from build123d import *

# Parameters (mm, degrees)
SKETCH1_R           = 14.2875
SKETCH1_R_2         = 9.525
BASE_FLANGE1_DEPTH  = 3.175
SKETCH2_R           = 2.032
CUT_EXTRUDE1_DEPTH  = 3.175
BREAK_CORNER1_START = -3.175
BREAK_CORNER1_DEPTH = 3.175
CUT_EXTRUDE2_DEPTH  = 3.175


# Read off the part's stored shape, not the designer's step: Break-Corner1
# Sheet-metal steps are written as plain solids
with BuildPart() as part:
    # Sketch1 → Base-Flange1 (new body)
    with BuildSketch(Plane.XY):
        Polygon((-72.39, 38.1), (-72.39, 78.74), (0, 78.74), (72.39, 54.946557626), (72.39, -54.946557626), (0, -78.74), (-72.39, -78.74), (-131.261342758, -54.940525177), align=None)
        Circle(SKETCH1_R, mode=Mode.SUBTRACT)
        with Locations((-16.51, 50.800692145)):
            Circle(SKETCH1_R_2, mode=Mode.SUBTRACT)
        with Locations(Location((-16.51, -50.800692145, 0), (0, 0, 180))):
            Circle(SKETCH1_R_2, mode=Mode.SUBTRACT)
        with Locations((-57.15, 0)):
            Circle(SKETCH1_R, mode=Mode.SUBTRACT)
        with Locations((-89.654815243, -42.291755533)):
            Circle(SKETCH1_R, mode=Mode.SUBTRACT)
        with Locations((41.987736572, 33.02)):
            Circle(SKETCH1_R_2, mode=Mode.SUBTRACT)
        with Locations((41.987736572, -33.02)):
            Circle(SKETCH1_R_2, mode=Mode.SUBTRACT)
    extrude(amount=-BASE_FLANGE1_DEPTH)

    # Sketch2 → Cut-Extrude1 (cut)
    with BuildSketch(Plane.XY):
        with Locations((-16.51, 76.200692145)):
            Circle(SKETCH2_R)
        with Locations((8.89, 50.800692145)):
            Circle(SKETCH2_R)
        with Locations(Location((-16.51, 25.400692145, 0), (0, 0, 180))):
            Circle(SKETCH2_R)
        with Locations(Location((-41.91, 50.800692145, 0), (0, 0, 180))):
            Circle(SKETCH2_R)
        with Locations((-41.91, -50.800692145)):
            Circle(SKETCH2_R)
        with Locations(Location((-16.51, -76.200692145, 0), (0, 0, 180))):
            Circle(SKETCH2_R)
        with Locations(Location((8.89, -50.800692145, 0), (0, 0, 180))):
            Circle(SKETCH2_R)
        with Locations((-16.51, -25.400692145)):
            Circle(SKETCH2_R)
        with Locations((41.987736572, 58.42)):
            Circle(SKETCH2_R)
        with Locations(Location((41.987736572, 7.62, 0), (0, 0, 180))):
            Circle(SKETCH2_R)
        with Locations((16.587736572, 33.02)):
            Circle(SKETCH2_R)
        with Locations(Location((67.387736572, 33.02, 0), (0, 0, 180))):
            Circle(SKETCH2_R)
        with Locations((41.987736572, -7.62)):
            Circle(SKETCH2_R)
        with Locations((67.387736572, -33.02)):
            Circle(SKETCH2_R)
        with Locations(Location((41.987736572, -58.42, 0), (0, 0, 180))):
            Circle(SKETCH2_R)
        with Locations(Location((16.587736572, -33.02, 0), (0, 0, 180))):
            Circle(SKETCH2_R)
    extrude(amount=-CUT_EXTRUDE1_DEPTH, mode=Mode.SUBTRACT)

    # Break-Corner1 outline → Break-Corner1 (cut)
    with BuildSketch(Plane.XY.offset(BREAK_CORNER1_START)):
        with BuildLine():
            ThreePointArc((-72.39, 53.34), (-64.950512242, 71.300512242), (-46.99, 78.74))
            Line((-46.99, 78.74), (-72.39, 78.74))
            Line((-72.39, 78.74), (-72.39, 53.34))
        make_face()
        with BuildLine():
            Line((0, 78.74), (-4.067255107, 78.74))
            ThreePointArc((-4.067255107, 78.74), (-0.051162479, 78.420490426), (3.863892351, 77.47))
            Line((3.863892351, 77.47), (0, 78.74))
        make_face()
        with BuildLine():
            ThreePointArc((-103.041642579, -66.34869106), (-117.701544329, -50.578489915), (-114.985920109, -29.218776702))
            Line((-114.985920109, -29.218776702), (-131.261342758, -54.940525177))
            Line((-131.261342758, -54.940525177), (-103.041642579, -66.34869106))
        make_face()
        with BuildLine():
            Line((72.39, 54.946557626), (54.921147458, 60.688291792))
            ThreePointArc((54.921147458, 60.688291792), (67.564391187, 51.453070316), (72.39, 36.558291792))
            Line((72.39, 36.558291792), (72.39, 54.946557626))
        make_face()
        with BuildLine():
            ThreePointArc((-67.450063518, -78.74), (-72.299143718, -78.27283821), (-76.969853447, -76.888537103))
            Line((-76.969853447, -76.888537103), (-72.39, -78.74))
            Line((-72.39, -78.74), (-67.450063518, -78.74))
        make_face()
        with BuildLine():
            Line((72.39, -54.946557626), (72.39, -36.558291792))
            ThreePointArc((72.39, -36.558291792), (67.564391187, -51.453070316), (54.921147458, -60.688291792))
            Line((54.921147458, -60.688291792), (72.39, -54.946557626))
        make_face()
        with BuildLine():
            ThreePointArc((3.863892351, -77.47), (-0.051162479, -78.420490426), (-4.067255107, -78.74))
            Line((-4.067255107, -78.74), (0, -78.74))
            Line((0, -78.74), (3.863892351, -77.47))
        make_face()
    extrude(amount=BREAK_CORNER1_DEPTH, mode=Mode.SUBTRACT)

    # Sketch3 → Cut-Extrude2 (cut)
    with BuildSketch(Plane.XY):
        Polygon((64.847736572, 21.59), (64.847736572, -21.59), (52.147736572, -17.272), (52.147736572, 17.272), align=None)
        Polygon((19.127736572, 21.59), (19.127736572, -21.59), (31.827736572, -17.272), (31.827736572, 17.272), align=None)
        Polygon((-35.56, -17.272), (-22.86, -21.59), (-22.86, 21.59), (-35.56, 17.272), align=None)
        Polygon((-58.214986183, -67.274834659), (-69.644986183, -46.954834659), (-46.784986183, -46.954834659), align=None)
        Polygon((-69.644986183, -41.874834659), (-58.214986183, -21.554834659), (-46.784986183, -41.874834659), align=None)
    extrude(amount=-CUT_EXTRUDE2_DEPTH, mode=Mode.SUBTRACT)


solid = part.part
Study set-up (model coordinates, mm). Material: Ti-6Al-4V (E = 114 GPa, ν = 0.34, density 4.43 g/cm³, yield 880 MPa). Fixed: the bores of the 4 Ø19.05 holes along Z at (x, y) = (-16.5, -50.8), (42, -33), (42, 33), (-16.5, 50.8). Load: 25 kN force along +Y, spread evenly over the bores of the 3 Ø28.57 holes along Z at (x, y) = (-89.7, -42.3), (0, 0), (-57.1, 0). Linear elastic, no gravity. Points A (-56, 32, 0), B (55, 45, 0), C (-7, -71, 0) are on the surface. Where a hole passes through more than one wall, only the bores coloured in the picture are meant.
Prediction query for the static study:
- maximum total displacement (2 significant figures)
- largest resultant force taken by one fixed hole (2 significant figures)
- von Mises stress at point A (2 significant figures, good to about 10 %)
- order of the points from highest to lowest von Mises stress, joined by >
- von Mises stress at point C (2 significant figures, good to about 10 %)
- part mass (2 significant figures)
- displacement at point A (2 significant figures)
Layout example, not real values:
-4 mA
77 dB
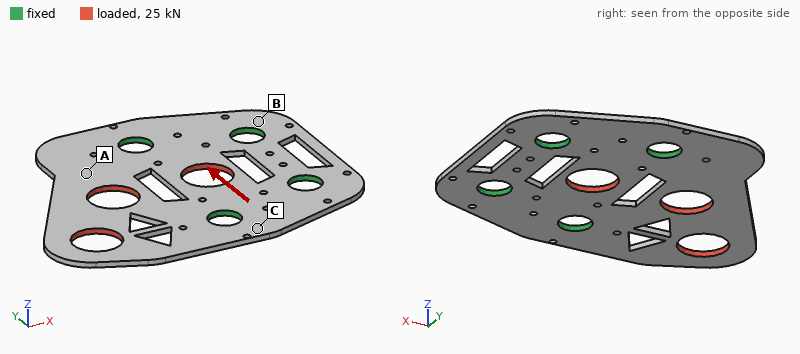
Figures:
0.19 mm
14 kN
91 MPa
A > C > B
49 MPa
260 g
0.076 mm
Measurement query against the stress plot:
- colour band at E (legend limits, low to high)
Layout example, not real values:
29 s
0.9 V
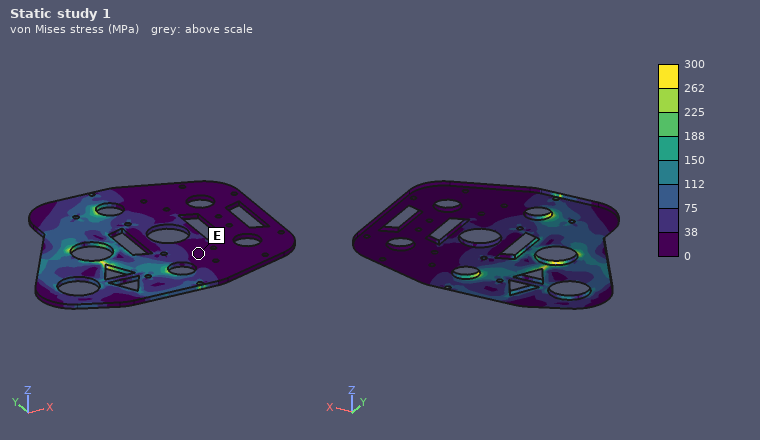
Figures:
0 to 38 MPa
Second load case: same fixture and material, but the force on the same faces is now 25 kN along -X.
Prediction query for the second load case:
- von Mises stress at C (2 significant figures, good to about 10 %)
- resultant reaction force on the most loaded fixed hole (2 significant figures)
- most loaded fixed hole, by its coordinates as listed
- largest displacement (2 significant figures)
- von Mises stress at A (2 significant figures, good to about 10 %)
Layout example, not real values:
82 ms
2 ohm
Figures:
25 MPa
12 kN
(-16.5, -50.8)
85 µm
50 MPa
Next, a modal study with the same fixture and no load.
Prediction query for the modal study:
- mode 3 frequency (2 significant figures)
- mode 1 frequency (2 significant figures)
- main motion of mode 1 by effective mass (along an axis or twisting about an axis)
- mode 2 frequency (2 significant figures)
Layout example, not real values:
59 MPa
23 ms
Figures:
1500 Hz
370 Hz
along Z
880 Hz
